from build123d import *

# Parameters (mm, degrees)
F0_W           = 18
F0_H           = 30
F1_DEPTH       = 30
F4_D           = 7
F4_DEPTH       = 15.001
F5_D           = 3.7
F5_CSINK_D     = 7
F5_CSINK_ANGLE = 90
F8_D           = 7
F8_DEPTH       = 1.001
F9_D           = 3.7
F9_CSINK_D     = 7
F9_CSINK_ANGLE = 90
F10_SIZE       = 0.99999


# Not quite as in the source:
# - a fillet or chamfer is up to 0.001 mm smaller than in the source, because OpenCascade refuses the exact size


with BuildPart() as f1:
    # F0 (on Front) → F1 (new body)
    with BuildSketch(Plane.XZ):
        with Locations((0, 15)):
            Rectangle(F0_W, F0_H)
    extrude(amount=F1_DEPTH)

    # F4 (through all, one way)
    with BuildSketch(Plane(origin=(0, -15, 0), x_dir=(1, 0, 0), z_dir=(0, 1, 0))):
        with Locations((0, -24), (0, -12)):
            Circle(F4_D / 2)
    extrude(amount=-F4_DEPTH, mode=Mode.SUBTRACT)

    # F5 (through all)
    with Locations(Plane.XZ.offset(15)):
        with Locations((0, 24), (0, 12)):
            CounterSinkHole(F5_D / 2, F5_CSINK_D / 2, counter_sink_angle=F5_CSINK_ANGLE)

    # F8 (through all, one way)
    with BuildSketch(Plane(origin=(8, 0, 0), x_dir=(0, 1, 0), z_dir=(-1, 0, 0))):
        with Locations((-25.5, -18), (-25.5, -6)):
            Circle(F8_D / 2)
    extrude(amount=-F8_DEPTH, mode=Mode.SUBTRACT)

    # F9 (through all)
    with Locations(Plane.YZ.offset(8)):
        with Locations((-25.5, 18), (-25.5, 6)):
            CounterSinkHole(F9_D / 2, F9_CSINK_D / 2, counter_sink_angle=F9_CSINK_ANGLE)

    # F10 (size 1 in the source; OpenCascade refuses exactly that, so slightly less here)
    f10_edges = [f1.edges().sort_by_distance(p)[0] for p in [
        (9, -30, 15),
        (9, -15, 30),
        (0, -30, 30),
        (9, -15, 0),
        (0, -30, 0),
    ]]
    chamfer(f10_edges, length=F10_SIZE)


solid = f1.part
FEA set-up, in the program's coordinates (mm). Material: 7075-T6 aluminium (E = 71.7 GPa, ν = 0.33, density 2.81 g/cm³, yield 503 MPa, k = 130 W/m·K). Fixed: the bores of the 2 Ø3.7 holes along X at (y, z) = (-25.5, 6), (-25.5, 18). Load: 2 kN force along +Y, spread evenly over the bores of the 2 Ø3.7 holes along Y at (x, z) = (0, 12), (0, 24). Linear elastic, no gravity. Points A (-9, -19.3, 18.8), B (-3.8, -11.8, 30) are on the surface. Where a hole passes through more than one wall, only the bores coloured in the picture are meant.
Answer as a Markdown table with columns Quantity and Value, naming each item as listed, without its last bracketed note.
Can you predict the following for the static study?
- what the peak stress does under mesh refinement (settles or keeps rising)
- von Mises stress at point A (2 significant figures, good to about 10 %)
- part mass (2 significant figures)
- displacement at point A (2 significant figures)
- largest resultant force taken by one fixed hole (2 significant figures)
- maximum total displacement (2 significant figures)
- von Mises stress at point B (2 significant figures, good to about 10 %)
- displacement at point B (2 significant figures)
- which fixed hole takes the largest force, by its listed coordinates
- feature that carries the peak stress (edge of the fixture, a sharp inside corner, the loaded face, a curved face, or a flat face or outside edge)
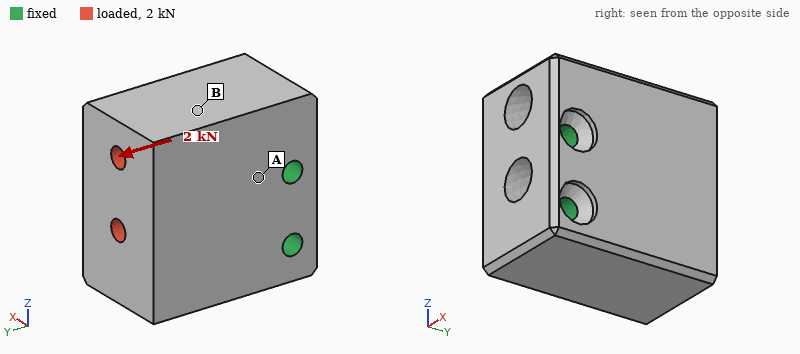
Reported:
| Quantity | Value |
|---|---|
| what the peak stress does under mesh refinement | keeps rising |
| von Mises stress at point A | 9.3 MPa |
| part mass | 40 g |
| displacement at point A | 1.1 µm |
| largest resultant force taken by one fixed hole | 1.8 kN |
| maximum total displacement | 4.9 µm |
| von Mises stress at point B | 4.1 MPa |
| displacement at point B | 3.7 µm |
| which fixed hole takes the largest force, by its listed coordinates | (-25.5, 18) |
| feature that carries the peak stress | edge of the fixture |
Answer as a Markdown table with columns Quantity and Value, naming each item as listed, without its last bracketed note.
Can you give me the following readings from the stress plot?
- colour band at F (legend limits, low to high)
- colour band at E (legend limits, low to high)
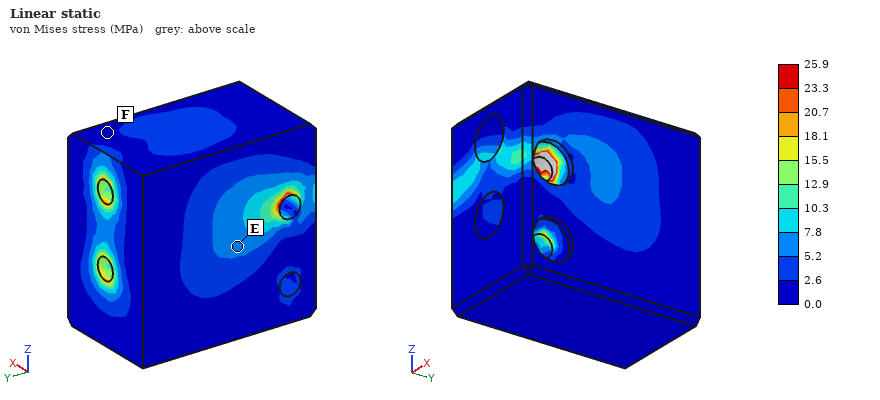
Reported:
| Quantity | Value |
|---|---|
| colour band at F | 0.0 to 2.6 MPa |
| colour band at E | 5.2 to 7.8 MPa |
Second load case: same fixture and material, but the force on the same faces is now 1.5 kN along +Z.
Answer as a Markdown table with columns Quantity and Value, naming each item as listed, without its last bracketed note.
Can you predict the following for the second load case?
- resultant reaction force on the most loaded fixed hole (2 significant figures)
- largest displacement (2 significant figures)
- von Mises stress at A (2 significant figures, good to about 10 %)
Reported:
| Quantity | Value |
|---|---|
| resultant reaction force on the most loaded fixed hole | 1.9 kN |
| largest displacement | 11 µm |
| von Mises stress at A | 11 MPa |
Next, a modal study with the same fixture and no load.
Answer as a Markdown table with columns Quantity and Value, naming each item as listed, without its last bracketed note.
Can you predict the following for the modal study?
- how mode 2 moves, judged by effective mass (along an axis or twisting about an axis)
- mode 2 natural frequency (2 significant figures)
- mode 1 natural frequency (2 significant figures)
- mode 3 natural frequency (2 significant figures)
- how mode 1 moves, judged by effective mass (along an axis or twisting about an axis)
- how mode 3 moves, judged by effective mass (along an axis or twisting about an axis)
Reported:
| Quantity | Value |
|---|---|
| how mode 2 moves, judged by effective mass | along Z |
| mode 2 natural frequency | 14 kHz |
| mode 1 natural frequency | 14 kHz |
| mode 3 natural frequency | 22 kHz |
| how mode 1 moves, judged by effective mass | along X |
| how mode 3 moves, judged by effective mass | twisting about Y |
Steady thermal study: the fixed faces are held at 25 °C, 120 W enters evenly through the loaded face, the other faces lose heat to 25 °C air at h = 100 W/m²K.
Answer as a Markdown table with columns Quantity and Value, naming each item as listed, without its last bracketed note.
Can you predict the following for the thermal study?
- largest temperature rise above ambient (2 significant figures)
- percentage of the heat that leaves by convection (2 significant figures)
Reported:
| Quantity | Value |
|---|---|
| largest temperature rise above ambient | 47 K |
| percentage of the heat that leaves by convection | 7.4 % |
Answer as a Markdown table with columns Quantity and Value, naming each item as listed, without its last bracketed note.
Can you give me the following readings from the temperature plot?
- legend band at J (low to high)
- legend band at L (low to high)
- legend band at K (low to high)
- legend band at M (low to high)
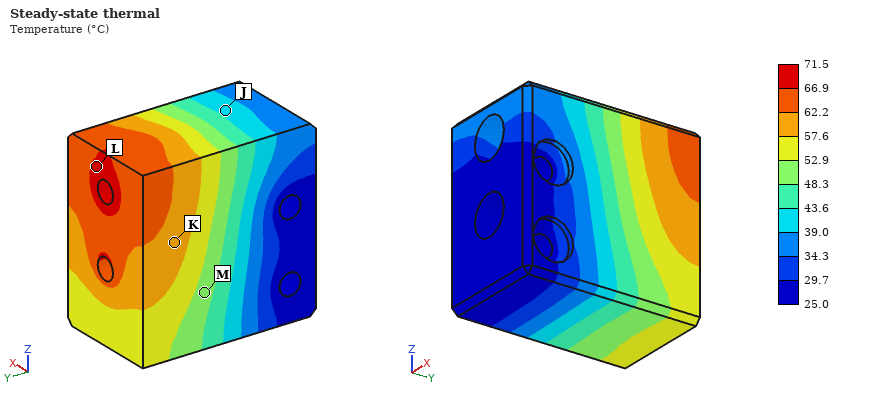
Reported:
| Quantity | Value |
|---|---|
| legend band at J | 39.0 to 43.6 °C |
| legend band at L | 66.9 to 71.5 °C |
| legend band at K | 57.6 to 62.2 °C |
| legend band at M | 48.3 to 52.9 °C |
